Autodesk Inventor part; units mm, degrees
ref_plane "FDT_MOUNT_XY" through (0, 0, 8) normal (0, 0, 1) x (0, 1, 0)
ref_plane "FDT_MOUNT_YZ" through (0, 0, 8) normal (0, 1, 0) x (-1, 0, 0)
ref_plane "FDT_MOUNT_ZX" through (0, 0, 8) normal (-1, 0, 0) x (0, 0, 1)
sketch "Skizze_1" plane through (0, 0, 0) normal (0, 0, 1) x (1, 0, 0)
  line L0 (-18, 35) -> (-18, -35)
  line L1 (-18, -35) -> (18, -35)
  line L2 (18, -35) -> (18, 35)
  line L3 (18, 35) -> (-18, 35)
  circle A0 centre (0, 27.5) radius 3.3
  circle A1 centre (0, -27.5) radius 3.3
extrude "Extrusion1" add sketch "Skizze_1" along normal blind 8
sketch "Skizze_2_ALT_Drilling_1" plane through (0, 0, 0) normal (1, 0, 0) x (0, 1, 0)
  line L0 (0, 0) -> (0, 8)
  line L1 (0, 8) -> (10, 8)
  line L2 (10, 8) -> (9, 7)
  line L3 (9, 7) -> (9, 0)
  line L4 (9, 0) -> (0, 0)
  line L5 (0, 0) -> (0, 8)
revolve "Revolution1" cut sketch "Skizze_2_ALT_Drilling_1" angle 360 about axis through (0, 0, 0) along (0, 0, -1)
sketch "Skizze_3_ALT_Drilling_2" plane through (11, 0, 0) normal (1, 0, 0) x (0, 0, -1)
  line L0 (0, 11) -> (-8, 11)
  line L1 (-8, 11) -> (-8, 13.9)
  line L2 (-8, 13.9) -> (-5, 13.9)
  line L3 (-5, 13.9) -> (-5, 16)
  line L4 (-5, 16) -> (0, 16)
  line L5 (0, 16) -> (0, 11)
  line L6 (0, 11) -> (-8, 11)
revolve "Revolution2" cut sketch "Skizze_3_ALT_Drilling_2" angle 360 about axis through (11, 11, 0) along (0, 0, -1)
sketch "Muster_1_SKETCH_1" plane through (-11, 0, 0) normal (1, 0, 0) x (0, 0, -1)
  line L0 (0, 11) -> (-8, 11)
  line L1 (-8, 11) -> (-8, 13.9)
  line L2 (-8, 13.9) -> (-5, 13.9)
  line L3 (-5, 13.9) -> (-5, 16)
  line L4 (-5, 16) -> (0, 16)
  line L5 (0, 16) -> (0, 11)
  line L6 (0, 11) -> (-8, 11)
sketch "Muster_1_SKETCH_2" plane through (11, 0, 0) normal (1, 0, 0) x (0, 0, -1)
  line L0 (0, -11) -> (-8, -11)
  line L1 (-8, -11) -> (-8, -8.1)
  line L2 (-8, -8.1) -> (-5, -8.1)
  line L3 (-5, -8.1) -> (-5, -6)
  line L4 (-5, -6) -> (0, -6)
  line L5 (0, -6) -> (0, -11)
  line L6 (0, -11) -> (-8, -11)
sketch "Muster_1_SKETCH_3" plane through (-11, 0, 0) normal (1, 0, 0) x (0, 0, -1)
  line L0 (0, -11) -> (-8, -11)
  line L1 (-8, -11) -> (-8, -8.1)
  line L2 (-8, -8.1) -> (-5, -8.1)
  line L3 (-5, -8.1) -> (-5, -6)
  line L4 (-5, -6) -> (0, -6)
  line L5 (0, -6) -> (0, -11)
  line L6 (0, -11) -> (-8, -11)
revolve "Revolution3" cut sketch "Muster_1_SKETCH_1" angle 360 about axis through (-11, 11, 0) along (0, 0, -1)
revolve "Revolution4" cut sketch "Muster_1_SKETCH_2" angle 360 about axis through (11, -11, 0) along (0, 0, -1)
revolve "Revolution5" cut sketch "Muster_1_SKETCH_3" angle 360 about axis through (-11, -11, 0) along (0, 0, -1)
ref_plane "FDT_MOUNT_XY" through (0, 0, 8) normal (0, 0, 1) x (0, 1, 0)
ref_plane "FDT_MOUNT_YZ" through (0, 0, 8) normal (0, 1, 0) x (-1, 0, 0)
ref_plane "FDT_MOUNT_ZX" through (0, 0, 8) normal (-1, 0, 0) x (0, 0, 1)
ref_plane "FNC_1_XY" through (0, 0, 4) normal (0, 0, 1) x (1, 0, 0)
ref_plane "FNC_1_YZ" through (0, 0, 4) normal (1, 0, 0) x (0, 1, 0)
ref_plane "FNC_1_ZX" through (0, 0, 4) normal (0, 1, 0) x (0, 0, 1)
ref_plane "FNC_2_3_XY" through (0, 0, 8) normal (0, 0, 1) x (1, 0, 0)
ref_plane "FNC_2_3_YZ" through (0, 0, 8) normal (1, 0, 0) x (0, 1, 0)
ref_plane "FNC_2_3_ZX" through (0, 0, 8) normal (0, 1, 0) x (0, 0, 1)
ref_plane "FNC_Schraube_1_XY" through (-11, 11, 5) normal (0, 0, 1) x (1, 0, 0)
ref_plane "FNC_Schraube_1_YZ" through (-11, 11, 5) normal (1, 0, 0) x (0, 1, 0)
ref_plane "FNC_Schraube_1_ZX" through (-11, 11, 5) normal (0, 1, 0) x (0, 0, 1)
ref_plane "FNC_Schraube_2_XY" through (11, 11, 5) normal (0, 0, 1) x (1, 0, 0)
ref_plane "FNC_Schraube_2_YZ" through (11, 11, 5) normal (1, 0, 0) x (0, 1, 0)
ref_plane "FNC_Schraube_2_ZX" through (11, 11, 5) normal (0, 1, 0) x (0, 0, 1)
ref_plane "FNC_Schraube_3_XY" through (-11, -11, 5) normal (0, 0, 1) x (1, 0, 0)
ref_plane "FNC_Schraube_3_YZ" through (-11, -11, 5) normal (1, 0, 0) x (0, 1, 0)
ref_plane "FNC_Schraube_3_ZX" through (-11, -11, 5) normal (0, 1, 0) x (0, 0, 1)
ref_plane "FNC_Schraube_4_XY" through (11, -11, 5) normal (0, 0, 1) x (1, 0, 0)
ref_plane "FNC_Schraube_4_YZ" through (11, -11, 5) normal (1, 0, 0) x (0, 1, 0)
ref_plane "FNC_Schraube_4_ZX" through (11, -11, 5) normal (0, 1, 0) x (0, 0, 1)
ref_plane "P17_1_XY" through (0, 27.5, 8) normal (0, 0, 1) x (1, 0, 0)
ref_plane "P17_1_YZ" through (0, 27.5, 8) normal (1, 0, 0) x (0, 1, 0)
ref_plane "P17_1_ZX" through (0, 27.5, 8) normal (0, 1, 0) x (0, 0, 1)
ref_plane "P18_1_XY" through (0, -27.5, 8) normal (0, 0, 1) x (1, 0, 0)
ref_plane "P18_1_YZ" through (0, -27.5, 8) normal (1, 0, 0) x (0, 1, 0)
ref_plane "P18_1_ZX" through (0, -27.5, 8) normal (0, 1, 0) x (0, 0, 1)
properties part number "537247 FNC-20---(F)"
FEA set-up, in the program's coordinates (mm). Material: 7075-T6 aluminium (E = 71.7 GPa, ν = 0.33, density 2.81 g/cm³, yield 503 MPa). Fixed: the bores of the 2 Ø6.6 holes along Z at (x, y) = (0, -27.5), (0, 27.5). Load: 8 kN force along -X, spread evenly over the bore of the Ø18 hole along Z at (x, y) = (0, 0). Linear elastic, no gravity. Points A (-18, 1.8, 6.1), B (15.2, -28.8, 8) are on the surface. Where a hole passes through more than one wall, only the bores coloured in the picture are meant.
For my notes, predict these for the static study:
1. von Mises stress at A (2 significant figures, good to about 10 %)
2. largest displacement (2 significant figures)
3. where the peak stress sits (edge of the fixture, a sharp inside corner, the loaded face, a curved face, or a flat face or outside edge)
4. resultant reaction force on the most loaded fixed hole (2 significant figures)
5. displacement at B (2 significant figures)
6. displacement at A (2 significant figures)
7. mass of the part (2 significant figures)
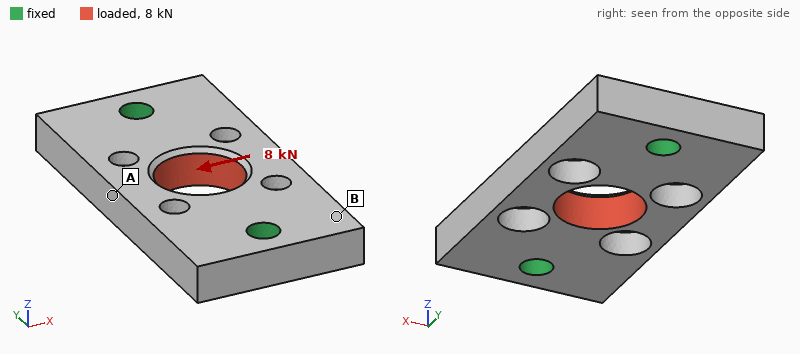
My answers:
73 MPa
41 µm
a curved face
4.0 kN
11 µm
33 µm
44 g
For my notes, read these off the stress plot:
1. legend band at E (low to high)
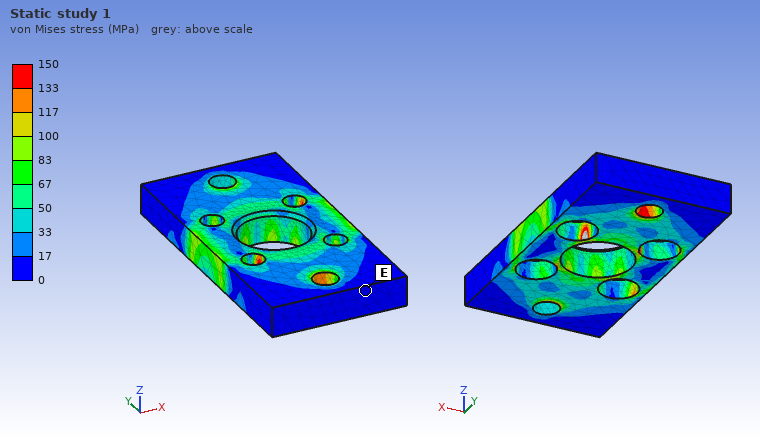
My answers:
0 to 17 MPa
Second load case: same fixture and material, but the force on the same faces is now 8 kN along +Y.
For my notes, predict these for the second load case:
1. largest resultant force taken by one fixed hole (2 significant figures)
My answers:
4.0 kN
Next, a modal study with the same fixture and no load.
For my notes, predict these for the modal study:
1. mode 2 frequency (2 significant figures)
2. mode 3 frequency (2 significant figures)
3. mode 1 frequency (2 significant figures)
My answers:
12 kHz
19 kHz
11 kHz
